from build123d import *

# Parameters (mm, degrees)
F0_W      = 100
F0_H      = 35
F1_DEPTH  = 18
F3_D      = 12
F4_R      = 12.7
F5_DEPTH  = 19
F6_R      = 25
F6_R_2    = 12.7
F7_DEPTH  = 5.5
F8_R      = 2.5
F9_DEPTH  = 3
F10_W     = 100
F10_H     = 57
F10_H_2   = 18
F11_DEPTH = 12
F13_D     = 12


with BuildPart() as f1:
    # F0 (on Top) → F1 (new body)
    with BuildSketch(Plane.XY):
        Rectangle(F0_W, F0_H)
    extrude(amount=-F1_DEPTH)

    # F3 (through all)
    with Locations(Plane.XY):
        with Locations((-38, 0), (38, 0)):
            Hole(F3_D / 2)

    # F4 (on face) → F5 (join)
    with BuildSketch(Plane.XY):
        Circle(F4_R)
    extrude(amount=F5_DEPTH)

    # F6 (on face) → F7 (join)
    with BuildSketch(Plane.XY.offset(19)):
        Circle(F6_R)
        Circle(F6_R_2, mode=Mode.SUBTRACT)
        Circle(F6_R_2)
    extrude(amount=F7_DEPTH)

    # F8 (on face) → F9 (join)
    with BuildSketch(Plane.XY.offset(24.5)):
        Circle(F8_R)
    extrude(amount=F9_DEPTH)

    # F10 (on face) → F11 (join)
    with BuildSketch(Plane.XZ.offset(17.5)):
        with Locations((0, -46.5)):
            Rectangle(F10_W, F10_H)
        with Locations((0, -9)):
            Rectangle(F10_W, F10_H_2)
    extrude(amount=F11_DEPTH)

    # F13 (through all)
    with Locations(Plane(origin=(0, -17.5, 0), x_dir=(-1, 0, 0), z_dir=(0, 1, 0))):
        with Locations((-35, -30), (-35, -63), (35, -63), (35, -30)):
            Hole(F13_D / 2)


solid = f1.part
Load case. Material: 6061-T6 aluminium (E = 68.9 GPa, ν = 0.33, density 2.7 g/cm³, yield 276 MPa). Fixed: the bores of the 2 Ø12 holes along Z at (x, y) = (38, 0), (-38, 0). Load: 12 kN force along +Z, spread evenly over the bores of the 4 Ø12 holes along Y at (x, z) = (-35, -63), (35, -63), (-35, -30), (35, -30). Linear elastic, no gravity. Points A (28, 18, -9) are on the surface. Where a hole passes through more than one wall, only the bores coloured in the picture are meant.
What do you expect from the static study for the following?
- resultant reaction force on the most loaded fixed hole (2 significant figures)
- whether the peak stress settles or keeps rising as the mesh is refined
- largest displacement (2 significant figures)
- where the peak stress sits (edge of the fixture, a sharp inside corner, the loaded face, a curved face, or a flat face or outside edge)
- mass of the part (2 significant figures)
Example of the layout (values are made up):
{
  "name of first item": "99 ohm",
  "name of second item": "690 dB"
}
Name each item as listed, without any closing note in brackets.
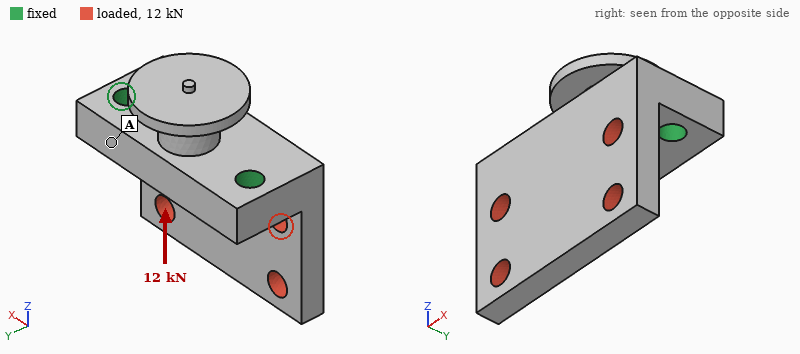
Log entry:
{
  "resultant reaction force on the most loaded fixed hole": "6.0 kN",
  "whether the peak stress settles or keeps rising as the mesh is refined": "keeps rising",
  "largest displacement": "95 µm",
  "where the peak stress sits": "edge of the fixture",
  "mass of the part": "440 g"
}
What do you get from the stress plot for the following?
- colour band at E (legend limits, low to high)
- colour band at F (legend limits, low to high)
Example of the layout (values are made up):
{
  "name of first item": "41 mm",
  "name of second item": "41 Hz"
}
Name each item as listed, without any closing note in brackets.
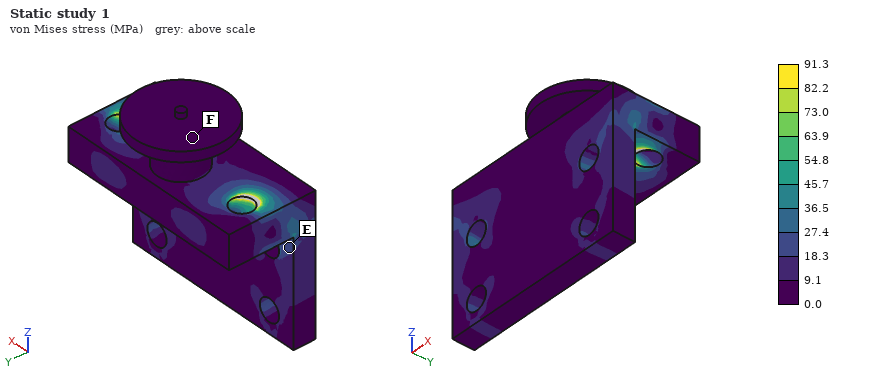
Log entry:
{
  "colour band at E": "18.3 to 27.4 MPa",
  "colour band at F": "0.0 to 9.1 MPa"
}
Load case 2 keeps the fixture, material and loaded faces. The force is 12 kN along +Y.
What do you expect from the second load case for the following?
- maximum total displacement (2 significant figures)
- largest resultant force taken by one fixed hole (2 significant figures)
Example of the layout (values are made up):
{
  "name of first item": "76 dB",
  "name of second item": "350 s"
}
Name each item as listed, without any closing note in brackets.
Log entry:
{
  "maximum total displacement": "0.67 mm",
  "largest resultant force taken by one fixed hole": "6.1 kN"
}
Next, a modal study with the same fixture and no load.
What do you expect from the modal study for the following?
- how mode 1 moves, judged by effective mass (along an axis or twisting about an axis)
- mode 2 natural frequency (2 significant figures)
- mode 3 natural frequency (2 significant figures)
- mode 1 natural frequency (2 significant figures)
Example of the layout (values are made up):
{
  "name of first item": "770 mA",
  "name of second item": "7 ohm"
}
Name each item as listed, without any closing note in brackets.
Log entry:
{
  "how mode 1 moves, judged by effective mass": "along Y",
  "mode 2 natural frequency": "3800 Hz",
  "mode 3 natural frequency": "5800 Hz",
  "mode 1 natural frequency": "2000 Hz"
}
